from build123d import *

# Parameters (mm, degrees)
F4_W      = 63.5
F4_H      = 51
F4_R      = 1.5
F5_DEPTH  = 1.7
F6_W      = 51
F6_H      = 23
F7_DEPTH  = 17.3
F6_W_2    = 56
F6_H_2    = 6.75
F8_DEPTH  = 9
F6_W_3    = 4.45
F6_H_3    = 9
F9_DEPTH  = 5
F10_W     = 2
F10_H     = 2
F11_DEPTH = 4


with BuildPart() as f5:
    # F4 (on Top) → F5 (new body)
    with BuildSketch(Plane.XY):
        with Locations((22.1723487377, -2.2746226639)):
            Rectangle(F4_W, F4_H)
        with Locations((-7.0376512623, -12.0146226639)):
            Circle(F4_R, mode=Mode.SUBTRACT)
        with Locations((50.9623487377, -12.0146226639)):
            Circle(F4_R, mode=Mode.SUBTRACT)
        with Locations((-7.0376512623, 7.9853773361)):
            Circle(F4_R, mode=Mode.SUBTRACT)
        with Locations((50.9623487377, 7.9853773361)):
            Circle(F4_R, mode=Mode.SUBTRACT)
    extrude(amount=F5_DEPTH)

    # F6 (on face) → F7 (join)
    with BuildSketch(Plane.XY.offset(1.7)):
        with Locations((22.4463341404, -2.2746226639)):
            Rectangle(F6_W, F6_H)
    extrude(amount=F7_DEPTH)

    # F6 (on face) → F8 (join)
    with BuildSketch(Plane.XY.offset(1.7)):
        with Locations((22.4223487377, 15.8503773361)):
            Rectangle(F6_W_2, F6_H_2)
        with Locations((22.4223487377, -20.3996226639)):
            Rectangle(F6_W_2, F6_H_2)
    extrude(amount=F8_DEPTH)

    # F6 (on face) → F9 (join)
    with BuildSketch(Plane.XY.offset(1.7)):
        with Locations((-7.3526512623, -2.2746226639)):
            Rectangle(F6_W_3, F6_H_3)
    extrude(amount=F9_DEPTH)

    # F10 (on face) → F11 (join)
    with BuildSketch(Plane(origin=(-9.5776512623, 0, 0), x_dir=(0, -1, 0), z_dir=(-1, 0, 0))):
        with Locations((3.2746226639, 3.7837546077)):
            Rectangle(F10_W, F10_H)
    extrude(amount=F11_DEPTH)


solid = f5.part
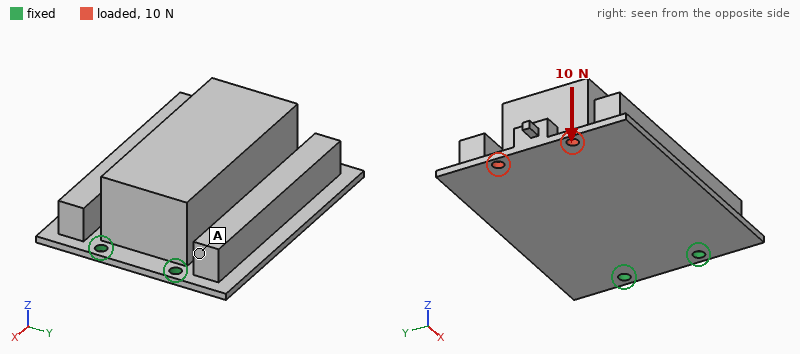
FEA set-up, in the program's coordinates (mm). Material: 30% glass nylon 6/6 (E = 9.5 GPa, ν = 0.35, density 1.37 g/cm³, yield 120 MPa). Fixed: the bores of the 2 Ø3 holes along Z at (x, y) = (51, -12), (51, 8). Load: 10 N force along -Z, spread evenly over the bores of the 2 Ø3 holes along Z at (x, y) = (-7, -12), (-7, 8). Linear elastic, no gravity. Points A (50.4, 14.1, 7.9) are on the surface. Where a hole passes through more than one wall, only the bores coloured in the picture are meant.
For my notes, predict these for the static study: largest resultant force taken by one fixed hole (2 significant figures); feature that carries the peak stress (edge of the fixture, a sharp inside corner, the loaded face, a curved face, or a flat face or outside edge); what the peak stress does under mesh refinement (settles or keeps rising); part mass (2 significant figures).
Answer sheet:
6.9 N
edge of the fixture
keeps rising
45 g
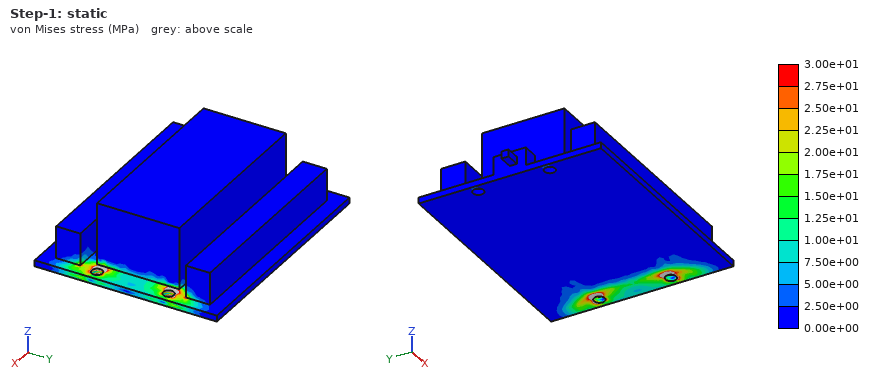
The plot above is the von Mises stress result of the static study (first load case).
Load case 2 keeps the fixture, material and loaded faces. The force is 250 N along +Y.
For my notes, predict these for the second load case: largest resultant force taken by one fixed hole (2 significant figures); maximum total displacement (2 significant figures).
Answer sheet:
680 N
0.30 mm
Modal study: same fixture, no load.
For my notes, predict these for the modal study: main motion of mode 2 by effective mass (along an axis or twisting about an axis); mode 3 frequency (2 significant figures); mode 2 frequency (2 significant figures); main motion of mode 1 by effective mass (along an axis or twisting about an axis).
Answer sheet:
along Y
1500 Hz
1300 Hz
along Z
